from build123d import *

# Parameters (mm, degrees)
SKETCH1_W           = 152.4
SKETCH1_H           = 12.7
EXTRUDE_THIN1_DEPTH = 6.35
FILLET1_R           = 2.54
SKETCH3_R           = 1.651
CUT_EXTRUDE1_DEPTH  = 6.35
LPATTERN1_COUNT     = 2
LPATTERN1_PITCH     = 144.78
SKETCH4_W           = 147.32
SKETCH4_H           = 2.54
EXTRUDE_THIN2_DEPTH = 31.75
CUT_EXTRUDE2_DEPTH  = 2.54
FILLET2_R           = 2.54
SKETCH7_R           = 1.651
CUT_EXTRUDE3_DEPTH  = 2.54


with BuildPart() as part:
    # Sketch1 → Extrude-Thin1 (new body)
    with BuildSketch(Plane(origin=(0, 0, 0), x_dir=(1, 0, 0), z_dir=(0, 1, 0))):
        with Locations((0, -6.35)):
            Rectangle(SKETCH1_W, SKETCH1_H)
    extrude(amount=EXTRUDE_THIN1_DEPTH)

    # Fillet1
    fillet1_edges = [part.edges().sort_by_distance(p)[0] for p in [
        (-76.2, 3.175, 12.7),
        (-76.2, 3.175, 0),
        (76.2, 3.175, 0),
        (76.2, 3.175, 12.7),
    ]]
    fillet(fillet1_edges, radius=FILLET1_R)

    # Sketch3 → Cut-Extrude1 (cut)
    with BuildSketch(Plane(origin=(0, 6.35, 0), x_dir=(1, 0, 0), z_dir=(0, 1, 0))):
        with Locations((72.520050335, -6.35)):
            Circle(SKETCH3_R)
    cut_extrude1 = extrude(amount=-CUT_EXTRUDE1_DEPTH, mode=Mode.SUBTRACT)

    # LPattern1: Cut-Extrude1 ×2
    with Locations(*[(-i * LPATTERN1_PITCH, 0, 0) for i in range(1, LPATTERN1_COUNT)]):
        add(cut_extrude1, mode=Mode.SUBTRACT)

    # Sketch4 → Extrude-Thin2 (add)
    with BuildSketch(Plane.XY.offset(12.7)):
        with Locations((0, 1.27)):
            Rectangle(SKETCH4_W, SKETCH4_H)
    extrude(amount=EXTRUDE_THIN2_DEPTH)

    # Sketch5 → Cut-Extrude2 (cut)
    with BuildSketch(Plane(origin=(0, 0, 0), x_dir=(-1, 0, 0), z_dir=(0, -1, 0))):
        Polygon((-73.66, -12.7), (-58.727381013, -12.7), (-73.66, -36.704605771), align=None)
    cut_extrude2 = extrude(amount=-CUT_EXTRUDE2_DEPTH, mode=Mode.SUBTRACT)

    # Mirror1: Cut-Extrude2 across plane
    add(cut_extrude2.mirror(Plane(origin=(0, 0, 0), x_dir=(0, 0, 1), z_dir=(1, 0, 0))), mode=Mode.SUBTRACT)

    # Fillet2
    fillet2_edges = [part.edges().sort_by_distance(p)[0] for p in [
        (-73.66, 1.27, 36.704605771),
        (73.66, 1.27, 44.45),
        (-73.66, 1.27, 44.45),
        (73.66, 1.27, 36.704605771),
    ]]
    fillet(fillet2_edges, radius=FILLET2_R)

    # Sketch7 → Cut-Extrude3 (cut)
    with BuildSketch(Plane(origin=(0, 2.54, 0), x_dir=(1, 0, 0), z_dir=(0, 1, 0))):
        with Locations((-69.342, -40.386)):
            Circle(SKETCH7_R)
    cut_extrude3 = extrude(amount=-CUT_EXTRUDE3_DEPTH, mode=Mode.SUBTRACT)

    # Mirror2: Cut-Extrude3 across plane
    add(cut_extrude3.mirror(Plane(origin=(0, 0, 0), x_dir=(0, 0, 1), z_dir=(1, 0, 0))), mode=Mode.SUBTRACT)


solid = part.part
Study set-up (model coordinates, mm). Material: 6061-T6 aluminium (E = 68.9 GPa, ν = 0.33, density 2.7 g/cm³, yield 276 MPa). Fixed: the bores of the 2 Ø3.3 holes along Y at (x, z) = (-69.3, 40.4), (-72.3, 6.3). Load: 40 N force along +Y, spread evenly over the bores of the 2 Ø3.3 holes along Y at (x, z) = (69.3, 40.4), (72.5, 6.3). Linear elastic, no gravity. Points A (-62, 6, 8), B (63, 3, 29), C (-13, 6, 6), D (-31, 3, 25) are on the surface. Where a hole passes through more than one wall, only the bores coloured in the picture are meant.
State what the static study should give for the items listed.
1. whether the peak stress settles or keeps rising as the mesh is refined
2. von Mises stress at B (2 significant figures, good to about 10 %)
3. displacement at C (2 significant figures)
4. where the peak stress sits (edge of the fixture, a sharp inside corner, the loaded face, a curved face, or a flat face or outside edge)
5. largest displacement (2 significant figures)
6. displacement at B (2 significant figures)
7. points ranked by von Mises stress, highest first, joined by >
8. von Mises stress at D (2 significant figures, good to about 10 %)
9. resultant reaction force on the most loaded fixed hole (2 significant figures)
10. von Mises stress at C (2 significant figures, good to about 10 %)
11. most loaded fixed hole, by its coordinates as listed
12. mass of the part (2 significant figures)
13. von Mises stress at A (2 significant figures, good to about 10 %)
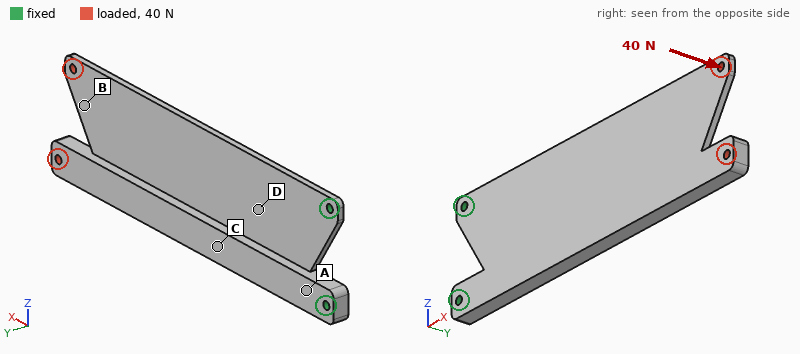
keeps rising
5.6 MPa
0.39 mm
edge of the fixture
1.8 mm
1.6 mm
A > C > D > B
10 MPa
76 N
33 MPa
(-72.3, 6.3)
62 g
57 MPa
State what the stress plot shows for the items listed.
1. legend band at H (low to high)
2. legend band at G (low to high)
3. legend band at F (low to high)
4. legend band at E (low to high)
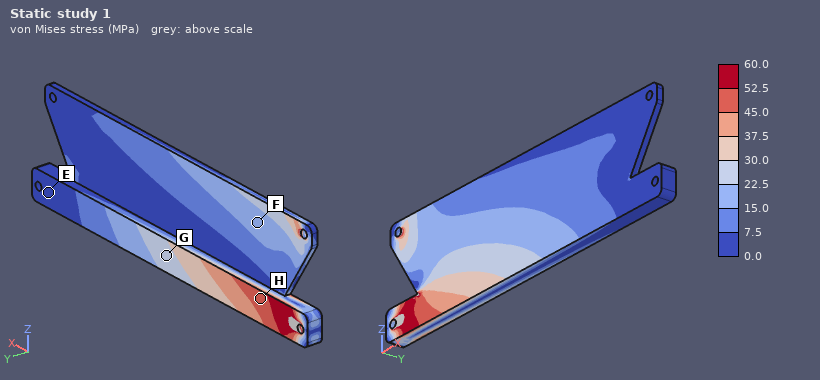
45.0 to 52.5 MPa
22.5 to 30.0 MPa
15.0 to 22.5 MPa
0.0 to 7.5 MPa
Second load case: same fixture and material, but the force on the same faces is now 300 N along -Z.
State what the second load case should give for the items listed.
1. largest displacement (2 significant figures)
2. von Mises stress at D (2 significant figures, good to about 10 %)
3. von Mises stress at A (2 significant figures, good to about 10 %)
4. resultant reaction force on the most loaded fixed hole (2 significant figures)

0.85 mm
15 MPa
11 MPa
1.2 kN
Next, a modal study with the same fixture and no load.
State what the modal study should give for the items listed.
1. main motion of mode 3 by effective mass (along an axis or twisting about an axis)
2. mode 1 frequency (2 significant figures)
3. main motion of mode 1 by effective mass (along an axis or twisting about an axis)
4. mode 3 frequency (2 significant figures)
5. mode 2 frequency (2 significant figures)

along Y
190 Hz
along Y
1200 Hz
940 Hz
